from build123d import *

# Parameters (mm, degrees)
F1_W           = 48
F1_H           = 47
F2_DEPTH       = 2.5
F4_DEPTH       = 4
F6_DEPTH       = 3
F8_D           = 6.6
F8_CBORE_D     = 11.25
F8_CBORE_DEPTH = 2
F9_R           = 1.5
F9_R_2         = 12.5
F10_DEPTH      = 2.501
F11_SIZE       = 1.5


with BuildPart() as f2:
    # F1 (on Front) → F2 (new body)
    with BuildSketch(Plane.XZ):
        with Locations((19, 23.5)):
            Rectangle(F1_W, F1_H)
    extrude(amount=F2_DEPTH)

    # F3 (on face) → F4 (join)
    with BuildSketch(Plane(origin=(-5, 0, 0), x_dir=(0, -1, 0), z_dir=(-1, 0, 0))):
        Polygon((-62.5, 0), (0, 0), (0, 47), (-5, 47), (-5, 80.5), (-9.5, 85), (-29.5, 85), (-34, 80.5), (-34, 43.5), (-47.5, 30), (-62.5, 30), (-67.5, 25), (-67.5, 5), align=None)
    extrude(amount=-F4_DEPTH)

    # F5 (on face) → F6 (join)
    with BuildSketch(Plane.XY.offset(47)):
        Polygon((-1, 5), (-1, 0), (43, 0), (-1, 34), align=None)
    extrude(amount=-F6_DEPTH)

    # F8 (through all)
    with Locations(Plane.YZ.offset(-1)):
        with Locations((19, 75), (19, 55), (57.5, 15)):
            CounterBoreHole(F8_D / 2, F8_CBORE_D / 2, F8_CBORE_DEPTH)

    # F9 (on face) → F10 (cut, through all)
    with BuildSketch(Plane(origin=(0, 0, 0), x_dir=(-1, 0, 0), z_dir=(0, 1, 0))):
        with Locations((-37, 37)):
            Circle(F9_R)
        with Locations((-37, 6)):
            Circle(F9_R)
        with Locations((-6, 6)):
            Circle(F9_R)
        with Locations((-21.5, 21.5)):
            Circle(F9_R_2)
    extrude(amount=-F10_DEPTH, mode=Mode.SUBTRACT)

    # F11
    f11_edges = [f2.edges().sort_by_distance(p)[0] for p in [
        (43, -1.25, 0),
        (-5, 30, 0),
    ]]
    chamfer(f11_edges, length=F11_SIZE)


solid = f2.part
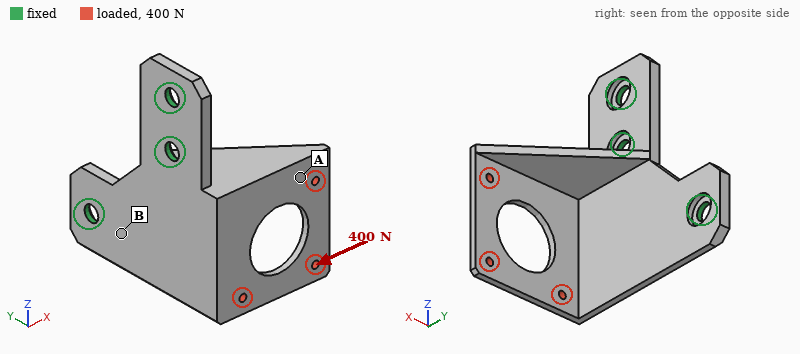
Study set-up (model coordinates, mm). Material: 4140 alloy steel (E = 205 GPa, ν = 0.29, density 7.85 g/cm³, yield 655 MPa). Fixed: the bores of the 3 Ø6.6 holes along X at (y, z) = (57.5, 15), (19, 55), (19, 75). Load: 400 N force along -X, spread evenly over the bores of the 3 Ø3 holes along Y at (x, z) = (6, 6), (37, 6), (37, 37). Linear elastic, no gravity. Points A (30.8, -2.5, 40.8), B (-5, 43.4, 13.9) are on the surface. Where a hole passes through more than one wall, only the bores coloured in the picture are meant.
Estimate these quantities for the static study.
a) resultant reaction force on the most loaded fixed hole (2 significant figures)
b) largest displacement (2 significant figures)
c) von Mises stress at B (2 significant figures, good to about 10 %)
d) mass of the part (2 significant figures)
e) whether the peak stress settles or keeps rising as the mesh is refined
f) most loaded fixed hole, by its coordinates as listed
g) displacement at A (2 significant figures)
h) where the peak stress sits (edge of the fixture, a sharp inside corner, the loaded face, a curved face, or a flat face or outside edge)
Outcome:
770 N
0.36 mm
53 MPa
160 g
keeps rising
(19, 55)
0.19 mm
edge of the fixture
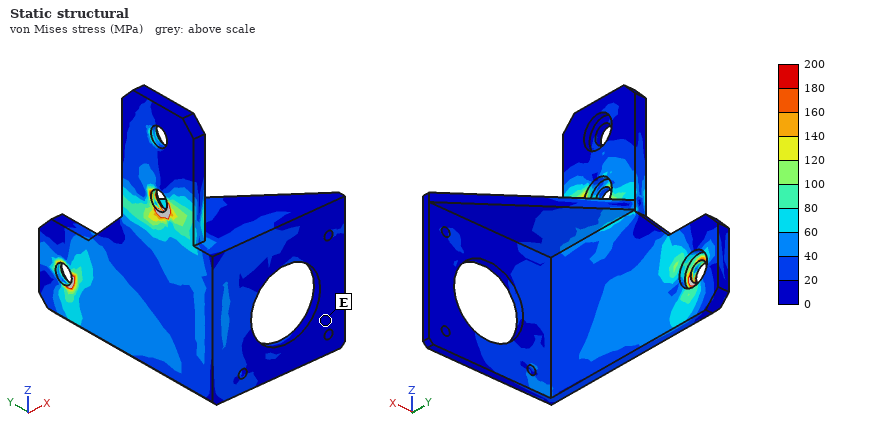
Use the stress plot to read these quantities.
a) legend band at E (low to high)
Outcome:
0 to 20 MPa
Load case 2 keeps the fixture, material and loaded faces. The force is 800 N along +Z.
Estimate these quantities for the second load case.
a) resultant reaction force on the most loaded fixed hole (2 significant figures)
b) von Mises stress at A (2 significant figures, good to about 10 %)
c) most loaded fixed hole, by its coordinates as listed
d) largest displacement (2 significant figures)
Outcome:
900 N
29 MPa
(19, 75)
0.56 mm
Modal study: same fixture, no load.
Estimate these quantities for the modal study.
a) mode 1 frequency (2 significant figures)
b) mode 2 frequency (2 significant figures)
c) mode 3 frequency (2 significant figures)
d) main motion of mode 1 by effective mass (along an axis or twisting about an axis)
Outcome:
880 Hz
1500 Hz
2600 Hz
along X
